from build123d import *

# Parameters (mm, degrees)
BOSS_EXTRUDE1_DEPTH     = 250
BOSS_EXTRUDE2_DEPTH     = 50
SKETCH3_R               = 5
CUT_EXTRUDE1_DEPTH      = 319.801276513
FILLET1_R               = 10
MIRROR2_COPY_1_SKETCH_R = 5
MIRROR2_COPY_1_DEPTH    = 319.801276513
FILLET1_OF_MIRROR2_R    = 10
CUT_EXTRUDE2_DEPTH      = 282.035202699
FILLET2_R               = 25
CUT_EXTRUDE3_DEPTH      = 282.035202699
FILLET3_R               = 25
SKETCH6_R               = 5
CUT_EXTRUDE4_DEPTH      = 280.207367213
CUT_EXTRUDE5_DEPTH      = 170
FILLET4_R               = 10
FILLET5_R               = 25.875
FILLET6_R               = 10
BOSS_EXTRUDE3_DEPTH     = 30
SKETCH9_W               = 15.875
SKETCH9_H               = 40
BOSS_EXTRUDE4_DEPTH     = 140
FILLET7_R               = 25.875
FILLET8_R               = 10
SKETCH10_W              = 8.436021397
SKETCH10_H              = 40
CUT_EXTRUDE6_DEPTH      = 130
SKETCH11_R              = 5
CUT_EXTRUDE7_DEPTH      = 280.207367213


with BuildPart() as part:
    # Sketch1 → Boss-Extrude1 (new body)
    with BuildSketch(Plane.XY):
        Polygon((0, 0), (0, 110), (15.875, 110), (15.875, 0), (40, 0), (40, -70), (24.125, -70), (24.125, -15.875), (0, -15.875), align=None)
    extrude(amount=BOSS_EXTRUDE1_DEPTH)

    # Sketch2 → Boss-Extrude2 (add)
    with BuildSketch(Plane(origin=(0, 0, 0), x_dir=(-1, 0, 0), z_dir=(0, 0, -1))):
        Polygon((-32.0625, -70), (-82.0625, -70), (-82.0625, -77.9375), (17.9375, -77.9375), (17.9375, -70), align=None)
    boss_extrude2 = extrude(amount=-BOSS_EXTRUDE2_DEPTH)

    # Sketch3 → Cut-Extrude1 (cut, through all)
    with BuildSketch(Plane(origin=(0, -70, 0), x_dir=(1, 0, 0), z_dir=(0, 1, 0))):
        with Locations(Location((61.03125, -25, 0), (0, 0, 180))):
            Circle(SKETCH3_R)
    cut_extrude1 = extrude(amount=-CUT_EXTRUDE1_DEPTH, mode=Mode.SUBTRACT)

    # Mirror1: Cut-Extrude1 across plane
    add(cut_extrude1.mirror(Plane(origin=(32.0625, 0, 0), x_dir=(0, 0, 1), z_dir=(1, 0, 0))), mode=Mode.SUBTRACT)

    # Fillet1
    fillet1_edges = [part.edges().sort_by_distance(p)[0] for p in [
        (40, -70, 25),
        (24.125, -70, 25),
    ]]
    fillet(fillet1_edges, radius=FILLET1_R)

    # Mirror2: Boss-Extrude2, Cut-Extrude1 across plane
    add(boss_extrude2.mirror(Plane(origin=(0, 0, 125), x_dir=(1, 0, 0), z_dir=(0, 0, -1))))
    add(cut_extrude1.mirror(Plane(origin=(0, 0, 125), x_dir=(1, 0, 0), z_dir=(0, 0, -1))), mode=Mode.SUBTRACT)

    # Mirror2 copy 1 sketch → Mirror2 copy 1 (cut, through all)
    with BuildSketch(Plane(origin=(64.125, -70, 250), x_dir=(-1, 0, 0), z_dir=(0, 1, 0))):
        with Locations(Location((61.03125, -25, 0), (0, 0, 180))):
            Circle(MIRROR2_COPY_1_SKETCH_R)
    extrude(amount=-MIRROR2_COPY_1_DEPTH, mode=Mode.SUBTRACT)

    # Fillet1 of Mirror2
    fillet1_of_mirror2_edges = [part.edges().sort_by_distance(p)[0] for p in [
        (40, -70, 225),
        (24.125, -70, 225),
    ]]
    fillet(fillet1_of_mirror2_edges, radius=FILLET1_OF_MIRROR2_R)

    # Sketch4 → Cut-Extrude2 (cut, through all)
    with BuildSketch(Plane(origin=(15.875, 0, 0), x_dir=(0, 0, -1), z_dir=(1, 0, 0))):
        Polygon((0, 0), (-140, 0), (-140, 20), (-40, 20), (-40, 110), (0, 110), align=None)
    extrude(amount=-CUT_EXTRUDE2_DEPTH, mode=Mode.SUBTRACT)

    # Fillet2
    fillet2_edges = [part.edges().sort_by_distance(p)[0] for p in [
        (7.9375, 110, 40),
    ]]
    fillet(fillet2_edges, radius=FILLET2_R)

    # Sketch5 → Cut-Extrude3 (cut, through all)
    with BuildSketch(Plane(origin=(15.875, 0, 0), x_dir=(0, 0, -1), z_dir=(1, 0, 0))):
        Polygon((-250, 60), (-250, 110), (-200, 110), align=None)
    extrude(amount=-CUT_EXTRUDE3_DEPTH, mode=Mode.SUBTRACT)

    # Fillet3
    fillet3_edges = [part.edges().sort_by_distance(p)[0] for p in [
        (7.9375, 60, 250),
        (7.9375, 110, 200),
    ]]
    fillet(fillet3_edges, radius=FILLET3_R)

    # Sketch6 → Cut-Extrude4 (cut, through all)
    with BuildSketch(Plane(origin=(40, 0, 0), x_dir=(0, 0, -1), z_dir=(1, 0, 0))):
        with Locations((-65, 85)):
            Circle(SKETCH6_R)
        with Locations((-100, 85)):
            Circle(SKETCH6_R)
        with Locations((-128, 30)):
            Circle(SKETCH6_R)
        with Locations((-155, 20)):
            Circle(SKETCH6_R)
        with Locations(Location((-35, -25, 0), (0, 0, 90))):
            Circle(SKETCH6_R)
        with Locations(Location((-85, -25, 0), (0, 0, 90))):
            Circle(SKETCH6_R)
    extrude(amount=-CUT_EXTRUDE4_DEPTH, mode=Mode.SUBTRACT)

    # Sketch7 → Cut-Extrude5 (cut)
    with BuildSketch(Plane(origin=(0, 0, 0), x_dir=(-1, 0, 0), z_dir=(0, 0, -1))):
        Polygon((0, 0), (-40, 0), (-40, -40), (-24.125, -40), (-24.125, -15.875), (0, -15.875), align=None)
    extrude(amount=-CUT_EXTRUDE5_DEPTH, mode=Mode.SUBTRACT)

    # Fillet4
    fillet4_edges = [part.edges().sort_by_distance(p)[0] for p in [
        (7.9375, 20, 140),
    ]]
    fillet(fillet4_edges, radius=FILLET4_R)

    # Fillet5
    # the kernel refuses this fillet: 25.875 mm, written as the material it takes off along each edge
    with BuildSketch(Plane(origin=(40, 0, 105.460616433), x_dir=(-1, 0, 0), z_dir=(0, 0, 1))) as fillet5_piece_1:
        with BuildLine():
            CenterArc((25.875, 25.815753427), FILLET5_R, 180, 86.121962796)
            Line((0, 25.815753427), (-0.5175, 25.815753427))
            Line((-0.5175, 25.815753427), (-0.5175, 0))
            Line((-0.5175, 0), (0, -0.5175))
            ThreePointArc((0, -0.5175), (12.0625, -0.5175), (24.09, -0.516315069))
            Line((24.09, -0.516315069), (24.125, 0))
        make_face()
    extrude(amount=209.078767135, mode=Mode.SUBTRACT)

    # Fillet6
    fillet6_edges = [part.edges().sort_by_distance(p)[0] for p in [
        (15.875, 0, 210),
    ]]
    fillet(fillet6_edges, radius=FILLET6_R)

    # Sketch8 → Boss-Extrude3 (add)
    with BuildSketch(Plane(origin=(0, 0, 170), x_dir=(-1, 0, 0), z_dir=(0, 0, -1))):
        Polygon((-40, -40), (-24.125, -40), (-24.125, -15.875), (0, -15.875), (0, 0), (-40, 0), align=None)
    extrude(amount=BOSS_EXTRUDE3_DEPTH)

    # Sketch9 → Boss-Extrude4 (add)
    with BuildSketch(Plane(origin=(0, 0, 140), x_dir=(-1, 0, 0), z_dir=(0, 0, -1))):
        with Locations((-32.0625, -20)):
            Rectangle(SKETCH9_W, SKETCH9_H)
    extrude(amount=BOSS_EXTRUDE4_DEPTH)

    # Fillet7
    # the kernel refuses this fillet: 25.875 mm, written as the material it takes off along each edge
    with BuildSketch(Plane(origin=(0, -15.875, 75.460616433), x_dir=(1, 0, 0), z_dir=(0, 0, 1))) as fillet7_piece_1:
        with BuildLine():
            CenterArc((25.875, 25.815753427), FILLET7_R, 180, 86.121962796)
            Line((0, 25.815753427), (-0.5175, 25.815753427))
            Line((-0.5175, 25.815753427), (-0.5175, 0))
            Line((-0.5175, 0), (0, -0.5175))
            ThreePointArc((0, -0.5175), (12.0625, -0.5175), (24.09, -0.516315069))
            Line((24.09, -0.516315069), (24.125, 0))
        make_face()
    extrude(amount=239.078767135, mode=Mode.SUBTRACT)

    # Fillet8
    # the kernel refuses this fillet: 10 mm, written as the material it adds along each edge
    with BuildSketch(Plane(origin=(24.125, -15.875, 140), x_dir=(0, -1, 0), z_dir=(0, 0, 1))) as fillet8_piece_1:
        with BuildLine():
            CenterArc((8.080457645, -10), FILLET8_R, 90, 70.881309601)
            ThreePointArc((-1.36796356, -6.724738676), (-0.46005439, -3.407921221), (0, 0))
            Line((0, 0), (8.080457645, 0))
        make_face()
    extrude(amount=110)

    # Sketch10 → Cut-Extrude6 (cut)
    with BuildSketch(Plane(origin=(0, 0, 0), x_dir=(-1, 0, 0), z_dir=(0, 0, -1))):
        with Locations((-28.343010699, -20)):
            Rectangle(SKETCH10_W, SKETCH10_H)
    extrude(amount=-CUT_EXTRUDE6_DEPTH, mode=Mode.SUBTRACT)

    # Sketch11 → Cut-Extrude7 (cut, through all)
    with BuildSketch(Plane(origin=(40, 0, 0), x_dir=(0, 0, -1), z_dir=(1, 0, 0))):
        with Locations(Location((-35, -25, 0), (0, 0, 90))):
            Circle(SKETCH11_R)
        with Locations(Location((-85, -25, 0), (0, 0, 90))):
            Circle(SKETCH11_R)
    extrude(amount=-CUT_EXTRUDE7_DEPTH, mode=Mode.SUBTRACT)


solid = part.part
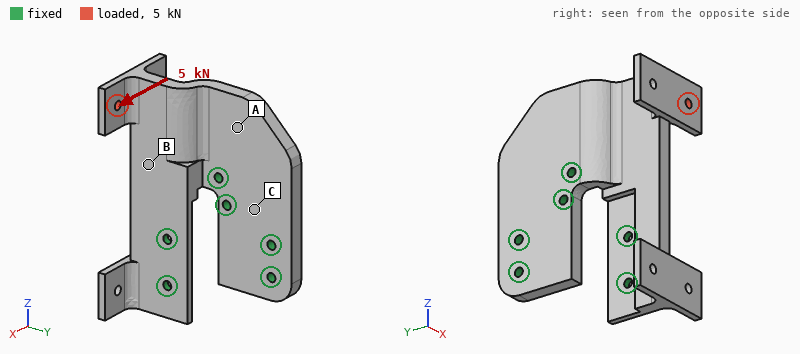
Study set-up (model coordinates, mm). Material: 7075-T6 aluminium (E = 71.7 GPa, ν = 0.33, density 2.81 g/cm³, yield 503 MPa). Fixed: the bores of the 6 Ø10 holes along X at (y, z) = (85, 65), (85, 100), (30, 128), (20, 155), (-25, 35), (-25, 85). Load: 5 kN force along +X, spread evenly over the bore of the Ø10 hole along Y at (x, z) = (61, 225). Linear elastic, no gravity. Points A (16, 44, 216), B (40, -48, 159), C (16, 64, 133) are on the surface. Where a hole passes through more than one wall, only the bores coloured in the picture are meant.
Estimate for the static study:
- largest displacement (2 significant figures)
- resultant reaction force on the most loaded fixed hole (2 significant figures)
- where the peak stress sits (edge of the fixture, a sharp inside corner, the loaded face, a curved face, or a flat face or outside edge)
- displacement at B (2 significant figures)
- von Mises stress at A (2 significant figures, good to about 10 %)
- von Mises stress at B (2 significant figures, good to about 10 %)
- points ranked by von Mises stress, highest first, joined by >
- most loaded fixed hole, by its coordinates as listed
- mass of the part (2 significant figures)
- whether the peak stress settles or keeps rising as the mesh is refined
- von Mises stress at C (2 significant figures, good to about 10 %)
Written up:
1.4 mm
13 kN
edge of the fixture
0.31 mm
37 MPa
55 MPa
B > A > C
(-25, 85)
1.8 kg
keeps rising
11 MPa
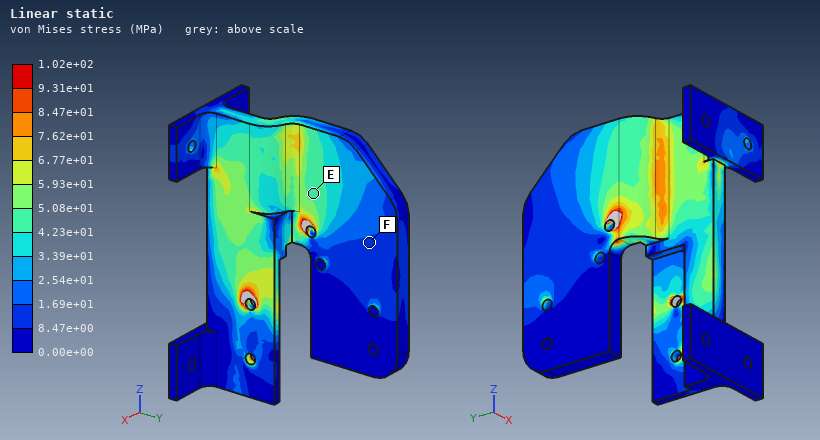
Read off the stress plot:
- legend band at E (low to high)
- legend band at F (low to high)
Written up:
4.23e+01 to 5.08e+01 MPa
8.47e+00 to 1.69e+01 MPa
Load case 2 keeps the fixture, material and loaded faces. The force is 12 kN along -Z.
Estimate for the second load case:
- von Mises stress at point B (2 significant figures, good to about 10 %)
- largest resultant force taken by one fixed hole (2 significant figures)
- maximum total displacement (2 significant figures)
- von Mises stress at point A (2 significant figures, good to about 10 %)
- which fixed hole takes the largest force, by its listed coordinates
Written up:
47 MPa
13 kN
0.76 mm
11 MPa
(-25, 85)
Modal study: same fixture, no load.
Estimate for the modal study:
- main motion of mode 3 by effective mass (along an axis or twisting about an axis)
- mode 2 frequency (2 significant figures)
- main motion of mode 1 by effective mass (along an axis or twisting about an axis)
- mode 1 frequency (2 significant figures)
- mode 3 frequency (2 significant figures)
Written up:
along X
1100 Hz
along X
770 Hz
1600 Hz
